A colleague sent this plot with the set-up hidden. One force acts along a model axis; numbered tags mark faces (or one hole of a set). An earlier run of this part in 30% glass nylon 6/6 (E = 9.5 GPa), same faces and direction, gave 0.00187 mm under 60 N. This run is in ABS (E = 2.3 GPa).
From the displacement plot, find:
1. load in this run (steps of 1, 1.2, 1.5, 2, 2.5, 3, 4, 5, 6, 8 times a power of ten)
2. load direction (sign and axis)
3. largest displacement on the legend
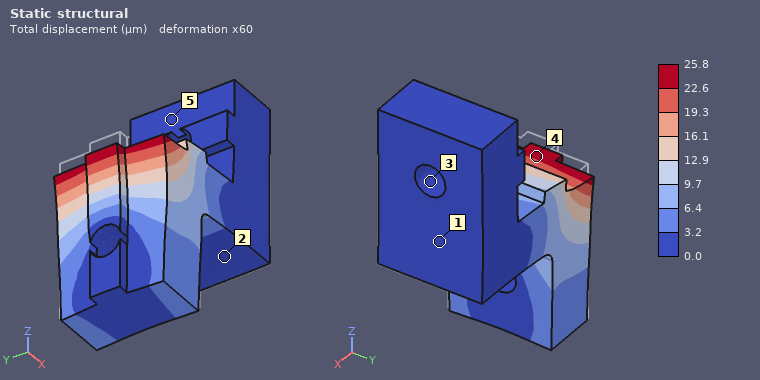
200 N
-Z
25.8 µm
